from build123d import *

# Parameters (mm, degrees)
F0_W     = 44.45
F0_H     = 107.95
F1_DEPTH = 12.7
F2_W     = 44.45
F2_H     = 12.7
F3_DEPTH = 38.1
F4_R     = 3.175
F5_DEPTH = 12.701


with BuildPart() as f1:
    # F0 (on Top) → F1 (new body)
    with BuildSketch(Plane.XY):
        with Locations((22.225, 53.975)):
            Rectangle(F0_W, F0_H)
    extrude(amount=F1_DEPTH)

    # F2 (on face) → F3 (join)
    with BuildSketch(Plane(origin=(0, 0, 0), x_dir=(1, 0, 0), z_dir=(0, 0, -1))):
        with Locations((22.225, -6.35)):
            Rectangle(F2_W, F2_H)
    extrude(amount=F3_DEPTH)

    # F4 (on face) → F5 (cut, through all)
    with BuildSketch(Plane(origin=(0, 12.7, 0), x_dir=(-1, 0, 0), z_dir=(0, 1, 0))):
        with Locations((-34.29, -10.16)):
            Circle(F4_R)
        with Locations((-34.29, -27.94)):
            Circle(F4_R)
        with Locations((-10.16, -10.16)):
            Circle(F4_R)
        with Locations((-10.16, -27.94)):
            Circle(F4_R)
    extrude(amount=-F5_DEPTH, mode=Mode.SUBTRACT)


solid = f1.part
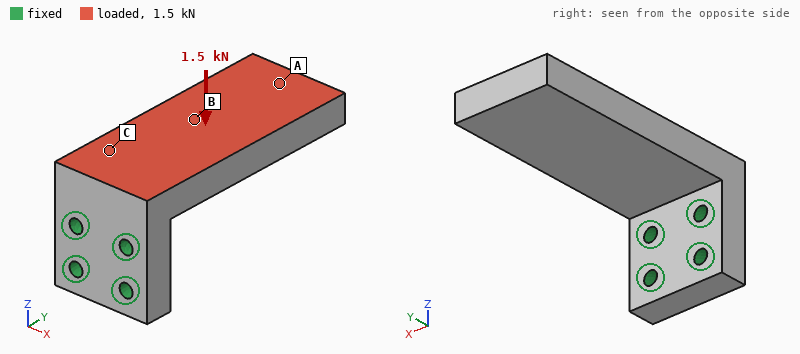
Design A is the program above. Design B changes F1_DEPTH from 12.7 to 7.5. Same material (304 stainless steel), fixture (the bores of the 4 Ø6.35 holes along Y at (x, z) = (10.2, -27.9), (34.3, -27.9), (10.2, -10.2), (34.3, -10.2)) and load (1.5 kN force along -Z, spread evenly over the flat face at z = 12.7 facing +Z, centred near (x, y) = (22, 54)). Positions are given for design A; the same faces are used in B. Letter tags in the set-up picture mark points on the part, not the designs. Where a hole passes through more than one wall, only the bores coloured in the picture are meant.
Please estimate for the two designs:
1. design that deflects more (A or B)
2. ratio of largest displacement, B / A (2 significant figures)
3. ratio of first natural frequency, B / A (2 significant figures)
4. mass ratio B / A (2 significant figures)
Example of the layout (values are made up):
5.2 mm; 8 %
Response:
B; 3.2; 0.73; 0.69
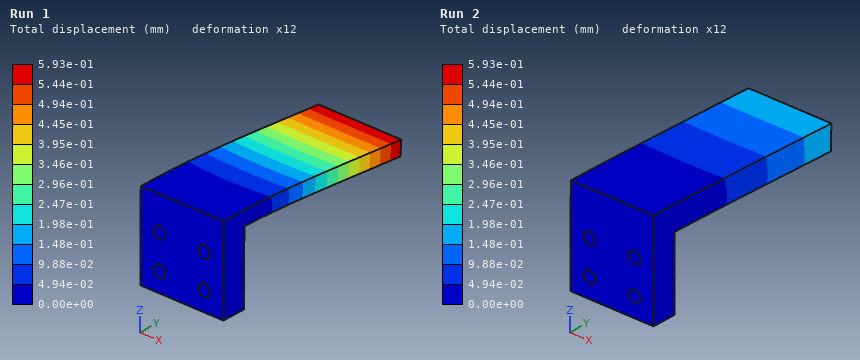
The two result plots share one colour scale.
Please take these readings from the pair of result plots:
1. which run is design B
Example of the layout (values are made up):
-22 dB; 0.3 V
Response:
Run 1
